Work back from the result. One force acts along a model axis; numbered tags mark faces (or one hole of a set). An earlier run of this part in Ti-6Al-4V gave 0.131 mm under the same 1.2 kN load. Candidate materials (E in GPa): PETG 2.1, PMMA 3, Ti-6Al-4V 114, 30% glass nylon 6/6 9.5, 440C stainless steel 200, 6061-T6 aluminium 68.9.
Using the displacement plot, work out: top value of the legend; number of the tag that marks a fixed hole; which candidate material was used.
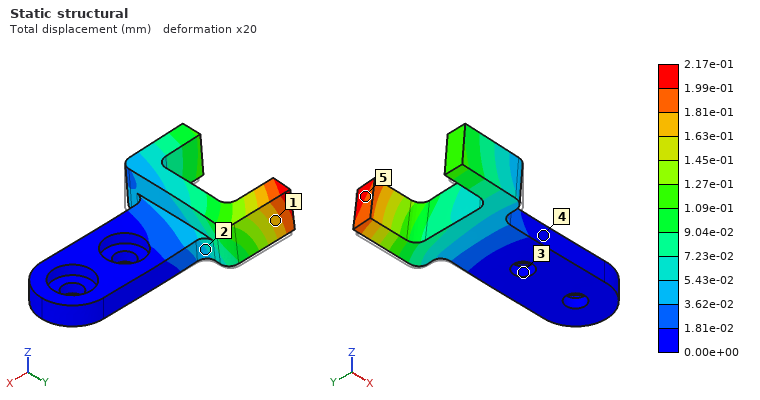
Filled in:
2.17e-01 mm
3
6061-T6 aluminium
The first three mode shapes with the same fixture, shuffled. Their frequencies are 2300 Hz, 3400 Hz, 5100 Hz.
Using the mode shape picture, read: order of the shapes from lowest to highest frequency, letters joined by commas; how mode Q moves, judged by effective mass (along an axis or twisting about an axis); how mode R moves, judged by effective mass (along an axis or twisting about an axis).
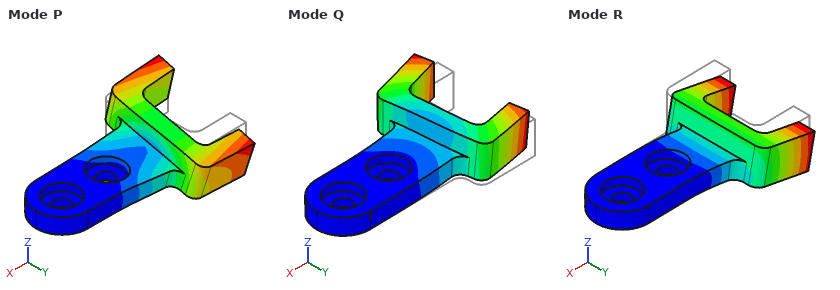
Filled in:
R, P, Q
along Y
along Z
